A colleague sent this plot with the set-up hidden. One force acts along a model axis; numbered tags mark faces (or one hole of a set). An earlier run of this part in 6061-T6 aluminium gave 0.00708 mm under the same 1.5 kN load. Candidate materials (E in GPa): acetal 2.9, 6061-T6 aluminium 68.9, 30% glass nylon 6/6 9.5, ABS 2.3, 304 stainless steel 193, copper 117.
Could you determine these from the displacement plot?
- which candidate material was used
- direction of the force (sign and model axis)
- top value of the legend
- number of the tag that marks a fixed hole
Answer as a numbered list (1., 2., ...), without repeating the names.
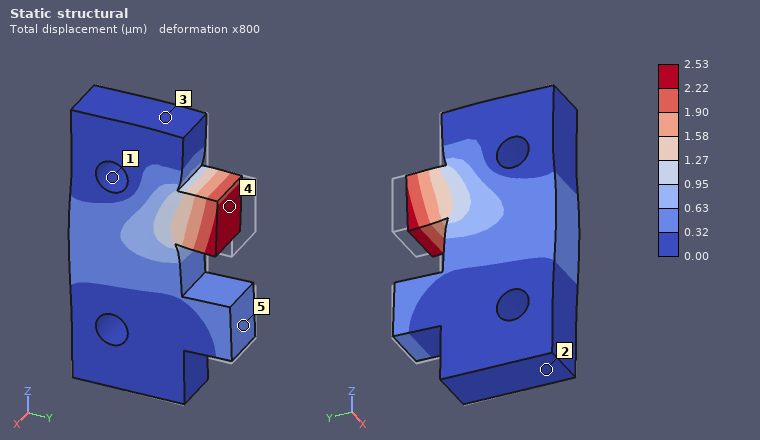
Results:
1. 304 stainless steel
2. -Y
3. 2.53 µm
4. 1
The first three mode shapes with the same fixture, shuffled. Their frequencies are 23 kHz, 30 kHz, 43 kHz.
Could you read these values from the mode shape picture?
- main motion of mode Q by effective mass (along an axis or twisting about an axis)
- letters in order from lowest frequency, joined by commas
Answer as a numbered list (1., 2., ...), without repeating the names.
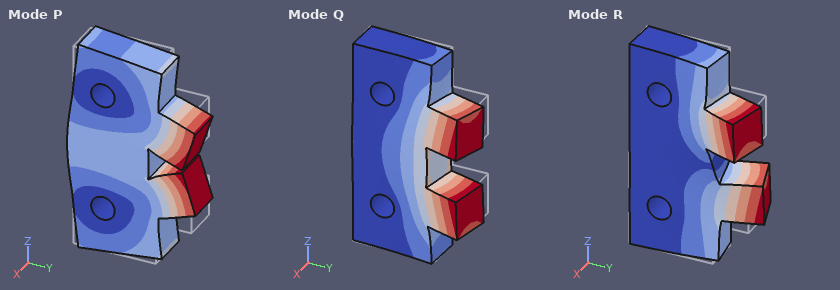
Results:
1. along X
2. Q, R, P
